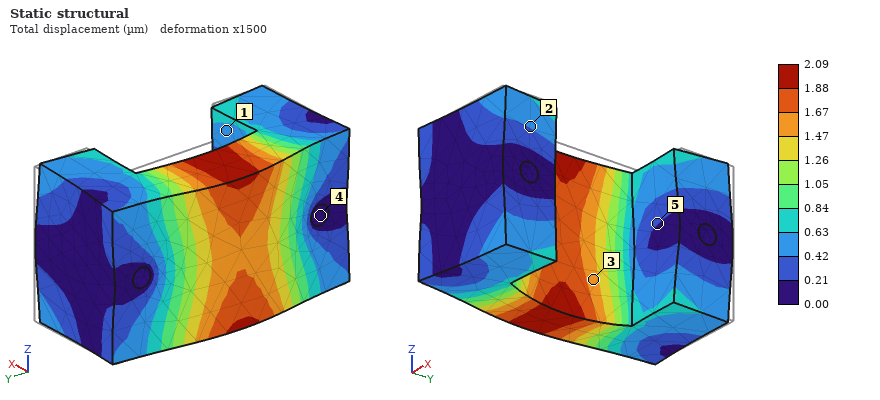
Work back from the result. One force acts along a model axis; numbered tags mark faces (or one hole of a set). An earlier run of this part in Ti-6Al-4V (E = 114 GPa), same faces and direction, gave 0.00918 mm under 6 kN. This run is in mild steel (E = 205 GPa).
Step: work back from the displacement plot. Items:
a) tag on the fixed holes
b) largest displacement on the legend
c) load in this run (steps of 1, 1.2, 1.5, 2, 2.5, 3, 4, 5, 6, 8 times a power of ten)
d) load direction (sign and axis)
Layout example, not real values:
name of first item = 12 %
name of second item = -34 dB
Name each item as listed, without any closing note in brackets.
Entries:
tag on the fixed holes = 4
largest displacement on the legend = 2.09 µm
load in this run = 2.5 kN
load direction = -X
